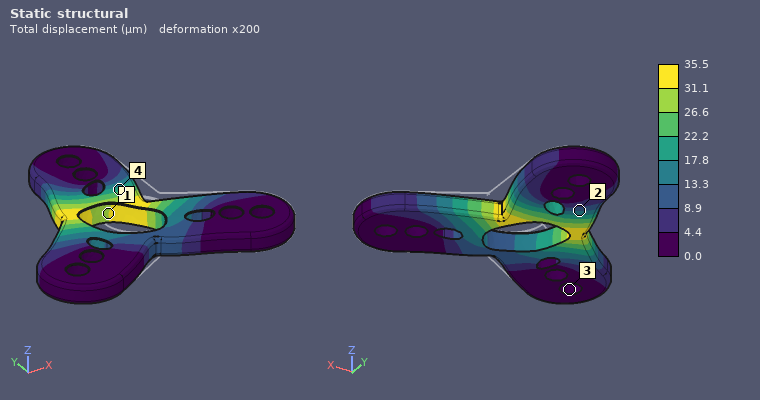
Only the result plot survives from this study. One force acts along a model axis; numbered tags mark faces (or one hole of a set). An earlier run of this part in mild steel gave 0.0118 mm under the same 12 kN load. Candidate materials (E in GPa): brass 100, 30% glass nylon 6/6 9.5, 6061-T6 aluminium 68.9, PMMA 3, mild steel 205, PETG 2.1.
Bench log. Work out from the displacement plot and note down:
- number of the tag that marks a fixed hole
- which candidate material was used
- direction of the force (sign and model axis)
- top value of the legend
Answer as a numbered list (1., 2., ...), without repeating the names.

1. 3
2. 6061-T6 aluminium
3. -X
4. 35.5 µm
